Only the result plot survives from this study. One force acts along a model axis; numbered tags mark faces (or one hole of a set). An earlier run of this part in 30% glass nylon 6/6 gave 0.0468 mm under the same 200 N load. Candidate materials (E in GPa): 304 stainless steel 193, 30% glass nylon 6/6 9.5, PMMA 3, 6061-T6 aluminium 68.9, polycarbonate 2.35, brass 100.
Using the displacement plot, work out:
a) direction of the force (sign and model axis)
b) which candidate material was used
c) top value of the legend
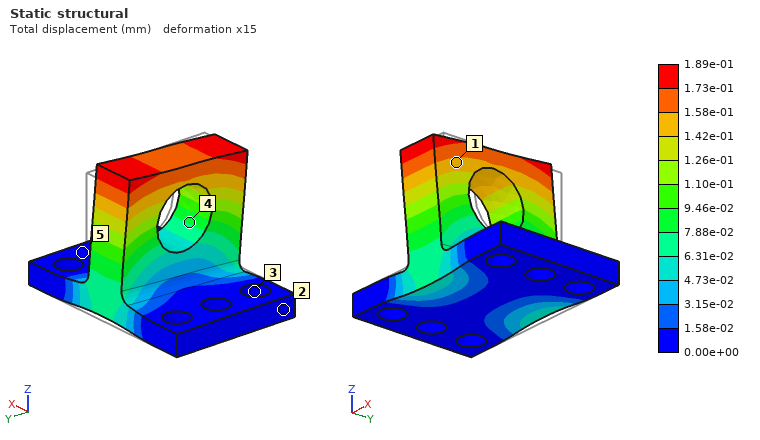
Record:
-Y
polycarbonate
1.89e-01 mm
